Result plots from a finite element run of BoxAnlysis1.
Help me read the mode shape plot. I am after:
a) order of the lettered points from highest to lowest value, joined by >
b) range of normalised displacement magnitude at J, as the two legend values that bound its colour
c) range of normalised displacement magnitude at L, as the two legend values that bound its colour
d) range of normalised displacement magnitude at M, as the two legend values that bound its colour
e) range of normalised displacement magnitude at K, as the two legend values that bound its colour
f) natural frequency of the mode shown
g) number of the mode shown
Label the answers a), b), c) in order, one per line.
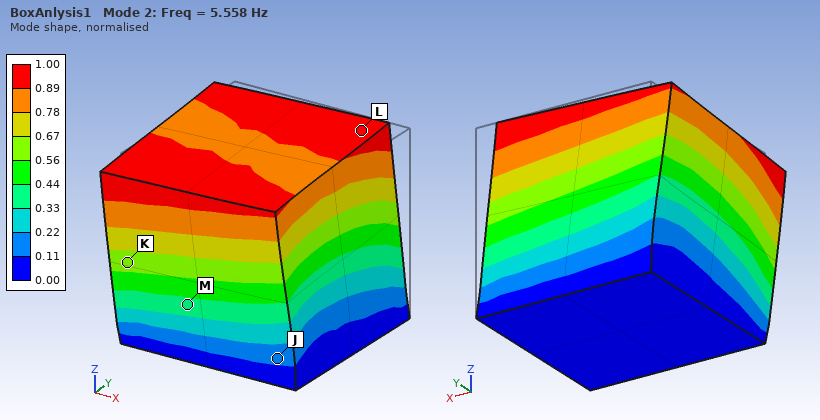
a) L > K > M > J
b) 0.11 to 0.22
c) 0.89 to 1.00
d) 0.33 to 0.44
e) 0.56 to 0.67
f) 5.558 Hz
g) 2
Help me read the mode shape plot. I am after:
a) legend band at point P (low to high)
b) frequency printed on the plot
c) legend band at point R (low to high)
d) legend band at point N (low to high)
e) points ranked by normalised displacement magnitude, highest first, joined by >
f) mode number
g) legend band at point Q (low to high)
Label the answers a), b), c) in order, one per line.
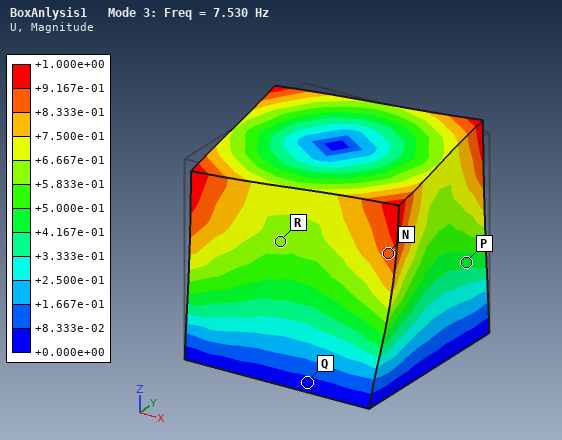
a) +4.167e-01 to +5.000e-01
b) 7.530 Hz
c) +5.833e-01 to +6.667e-01
d) +8.333e-01 to +9.167e-01
e) N > R > P > Q
f) 3
g) +0.000e+00 to +8.333e-02
